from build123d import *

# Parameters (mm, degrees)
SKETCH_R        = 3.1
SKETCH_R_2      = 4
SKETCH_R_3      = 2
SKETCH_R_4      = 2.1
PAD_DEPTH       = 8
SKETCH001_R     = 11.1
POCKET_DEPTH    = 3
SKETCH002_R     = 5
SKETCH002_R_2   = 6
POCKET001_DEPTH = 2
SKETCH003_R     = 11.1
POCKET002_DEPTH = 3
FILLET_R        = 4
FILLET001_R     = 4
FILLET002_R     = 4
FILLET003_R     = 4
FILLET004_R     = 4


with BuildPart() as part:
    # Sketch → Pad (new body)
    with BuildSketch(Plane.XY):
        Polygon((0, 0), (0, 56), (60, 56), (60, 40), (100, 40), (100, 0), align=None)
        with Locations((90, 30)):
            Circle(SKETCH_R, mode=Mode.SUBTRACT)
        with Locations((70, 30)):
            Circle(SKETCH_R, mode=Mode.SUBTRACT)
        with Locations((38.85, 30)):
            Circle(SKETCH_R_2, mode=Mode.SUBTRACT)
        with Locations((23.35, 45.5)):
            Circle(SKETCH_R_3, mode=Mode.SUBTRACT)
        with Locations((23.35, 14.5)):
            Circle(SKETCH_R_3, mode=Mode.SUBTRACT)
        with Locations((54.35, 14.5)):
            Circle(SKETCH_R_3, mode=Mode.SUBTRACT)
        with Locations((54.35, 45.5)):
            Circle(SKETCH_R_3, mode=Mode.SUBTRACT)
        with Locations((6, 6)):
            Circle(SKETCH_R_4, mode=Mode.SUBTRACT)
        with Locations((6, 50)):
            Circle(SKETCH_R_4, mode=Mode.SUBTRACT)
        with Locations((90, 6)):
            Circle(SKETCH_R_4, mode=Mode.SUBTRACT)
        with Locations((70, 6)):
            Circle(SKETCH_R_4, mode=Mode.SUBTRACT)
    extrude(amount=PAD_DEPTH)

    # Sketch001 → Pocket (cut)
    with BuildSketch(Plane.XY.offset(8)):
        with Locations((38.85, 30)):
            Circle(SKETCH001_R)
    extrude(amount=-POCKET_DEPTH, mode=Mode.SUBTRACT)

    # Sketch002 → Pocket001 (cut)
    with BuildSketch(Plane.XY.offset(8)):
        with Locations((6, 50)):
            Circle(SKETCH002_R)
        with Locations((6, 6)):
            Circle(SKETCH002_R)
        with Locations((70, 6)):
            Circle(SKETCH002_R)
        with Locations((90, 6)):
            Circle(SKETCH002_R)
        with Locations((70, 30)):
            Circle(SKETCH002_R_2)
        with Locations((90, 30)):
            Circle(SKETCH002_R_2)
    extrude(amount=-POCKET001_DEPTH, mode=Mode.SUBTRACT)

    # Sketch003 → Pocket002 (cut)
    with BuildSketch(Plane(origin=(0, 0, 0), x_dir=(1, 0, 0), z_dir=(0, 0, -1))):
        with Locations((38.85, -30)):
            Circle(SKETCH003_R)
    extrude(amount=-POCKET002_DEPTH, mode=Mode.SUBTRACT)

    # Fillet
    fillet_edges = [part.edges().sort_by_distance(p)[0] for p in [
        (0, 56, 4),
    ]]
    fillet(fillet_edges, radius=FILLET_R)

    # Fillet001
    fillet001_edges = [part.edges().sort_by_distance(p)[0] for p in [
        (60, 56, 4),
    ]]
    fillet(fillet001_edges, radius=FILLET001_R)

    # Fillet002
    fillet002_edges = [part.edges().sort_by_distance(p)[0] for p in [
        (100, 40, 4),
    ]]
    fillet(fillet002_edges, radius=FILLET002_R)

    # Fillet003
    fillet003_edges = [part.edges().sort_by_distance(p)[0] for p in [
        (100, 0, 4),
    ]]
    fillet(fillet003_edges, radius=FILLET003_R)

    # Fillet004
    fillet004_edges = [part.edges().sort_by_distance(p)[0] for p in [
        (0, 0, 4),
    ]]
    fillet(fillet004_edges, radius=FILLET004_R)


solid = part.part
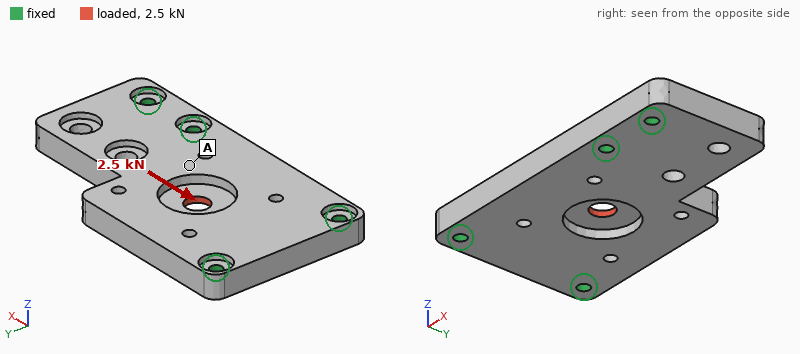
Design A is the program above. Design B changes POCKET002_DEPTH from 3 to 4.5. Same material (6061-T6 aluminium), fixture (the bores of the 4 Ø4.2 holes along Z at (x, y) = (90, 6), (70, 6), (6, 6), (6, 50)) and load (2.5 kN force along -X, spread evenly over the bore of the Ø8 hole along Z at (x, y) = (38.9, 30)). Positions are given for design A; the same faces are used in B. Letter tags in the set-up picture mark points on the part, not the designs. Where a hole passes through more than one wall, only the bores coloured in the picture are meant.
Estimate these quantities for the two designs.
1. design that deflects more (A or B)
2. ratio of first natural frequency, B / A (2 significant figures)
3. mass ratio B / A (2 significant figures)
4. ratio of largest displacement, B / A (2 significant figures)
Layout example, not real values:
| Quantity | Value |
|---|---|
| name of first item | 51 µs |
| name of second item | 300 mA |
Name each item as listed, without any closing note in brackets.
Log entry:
| Quantity | Value |
|---|---|
| design that deflects more | B |
| ratio of first natural frequency, B / A | 1.0 |
| mass ratio B / A | 0.99 |
| ratio of largest displacement, B / A | 2.5 |
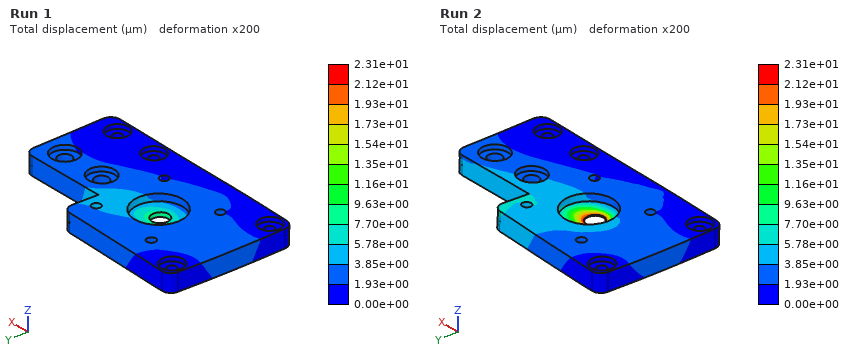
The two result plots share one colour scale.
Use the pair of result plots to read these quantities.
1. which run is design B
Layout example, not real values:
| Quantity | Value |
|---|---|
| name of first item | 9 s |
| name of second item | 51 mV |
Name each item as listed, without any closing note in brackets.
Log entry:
| Quantity | Value |
|---|---|
| which run is design B | Run 2 |
